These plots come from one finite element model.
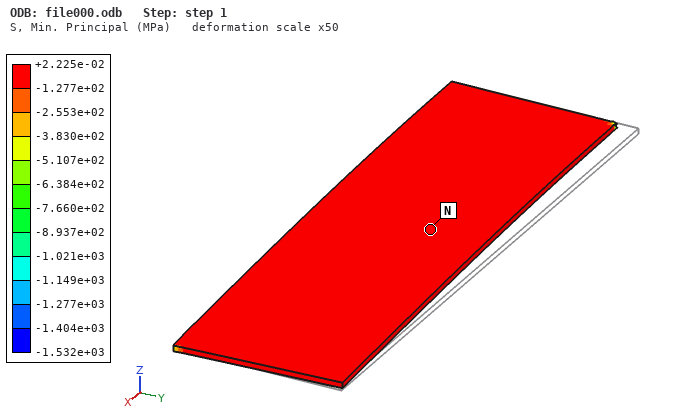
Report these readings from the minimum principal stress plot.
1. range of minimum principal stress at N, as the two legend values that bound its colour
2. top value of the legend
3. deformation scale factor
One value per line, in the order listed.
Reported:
-1.277e+02 to +2.225e-02 MPa
+2.225e-02 MPa
50
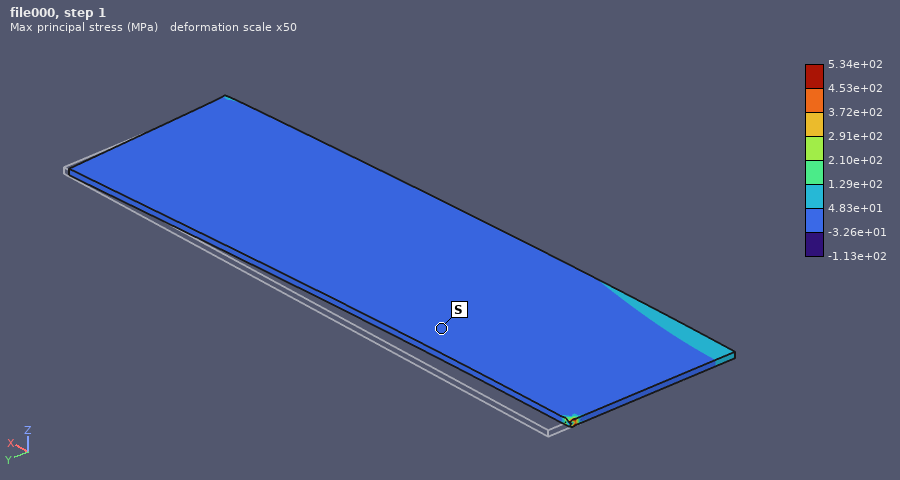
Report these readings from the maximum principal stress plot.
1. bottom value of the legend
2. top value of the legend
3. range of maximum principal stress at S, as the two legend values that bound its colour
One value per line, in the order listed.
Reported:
-1.13e+02 MPa
5.34e+02 MPa
-3.26e+01 to 4.83e+01 MPa
